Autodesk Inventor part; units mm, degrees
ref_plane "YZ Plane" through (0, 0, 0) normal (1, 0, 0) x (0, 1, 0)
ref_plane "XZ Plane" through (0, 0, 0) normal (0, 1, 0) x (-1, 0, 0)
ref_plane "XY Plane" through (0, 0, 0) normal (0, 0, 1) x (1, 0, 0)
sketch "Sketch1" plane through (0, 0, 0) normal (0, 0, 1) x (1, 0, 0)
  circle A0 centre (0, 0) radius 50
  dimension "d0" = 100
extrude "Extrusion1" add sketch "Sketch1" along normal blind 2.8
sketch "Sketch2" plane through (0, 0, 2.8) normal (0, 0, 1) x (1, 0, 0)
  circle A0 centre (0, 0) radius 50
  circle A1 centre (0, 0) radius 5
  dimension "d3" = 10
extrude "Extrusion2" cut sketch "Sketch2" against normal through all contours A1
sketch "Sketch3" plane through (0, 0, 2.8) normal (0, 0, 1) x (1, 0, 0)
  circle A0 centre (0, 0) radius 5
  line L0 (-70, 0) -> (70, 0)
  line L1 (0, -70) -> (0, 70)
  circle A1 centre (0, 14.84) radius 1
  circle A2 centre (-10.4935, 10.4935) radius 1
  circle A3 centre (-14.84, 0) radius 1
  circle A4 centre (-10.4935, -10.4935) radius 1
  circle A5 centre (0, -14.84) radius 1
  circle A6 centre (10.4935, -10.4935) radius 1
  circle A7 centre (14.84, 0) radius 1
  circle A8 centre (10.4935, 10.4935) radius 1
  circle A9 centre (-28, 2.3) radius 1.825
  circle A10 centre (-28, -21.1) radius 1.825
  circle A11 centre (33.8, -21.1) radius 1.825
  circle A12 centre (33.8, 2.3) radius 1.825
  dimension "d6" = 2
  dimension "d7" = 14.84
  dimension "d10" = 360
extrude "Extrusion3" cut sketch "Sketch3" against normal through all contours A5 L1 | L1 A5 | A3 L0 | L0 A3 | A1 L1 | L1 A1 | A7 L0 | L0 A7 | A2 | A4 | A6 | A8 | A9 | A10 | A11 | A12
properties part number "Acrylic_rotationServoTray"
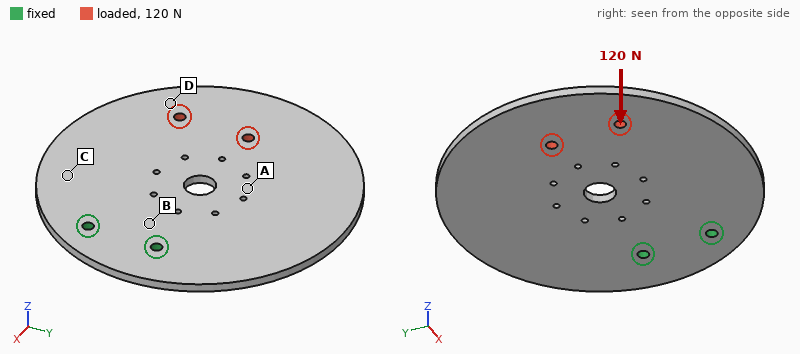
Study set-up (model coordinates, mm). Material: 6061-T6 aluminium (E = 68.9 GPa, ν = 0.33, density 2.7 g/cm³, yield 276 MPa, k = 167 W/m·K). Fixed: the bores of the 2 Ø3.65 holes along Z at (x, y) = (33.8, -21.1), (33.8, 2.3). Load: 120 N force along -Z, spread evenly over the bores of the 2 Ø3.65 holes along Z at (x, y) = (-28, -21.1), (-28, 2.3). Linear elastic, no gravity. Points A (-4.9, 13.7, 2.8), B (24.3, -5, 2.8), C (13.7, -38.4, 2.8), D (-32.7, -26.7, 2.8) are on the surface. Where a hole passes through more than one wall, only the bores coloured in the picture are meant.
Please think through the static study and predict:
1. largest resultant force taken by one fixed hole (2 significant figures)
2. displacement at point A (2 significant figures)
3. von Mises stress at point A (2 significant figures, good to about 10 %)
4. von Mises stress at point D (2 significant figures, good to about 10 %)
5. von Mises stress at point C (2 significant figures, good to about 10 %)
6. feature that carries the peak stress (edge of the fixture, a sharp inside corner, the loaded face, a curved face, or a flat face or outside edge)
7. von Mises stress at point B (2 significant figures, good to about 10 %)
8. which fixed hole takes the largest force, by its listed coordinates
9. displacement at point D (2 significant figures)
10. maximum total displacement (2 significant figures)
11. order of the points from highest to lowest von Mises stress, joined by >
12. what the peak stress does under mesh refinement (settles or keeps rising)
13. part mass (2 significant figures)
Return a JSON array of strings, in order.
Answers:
["65 N", "0.52 mm", "25 MPa", "9.4 MPa", "41 MPa", "edge of the fixture", "67 MPa", "(33.8, -21.1)", "1.2 mm", "1.6 mm", "B > C > A > D", "keeps rising", "58 g"]
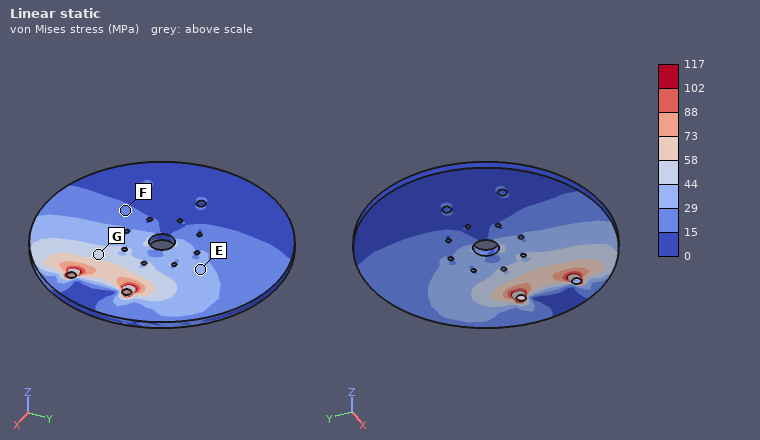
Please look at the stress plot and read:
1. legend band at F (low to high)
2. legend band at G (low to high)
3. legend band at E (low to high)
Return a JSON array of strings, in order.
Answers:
["15 to 29 MPa", "44 to 58 MPa", "29 to 44 MPa"]
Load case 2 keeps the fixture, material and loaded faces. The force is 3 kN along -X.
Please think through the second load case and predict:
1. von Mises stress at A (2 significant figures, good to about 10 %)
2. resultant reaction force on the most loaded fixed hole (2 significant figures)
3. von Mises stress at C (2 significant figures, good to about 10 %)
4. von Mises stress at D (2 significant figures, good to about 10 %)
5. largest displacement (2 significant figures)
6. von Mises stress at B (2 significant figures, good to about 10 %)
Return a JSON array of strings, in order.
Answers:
["14 MPa", "1.5 kN", "8.5 MPa", "15 MPa", "25 µm", "18 MPa"]
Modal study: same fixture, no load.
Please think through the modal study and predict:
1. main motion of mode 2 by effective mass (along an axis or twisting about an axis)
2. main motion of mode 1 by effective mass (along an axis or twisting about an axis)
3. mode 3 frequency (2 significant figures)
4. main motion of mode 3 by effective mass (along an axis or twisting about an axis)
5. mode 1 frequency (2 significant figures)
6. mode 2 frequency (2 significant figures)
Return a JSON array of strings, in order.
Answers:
["twisting about X", "along Z", "1400 Hz", "along Z", "340 Hz", "660 Hz"]
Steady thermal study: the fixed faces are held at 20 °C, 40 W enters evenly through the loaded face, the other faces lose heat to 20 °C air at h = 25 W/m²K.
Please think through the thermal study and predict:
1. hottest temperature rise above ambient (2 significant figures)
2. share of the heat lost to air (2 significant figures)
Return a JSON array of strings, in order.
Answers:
["71 K", "34 %"]
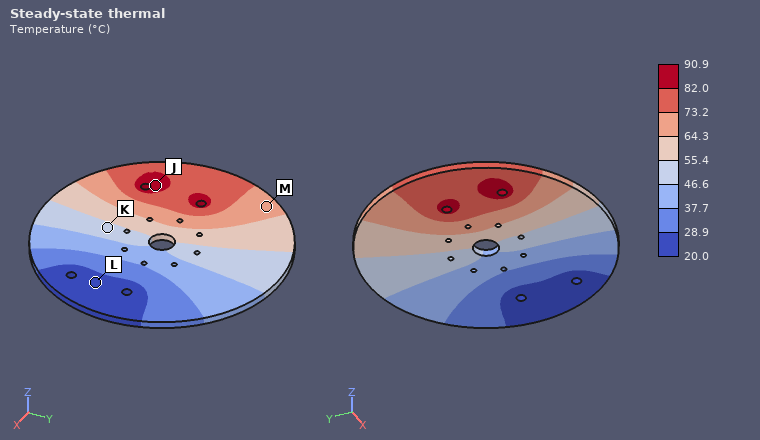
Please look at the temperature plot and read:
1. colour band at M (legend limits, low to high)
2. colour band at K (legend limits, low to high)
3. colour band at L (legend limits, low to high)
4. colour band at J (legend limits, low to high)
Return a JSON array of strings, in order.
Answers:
["64.3 to 73.2 °C", "46.6 to 55.4 °C", "20.0 to 28.9 °C", "82.0 to 90.9 °C"]
